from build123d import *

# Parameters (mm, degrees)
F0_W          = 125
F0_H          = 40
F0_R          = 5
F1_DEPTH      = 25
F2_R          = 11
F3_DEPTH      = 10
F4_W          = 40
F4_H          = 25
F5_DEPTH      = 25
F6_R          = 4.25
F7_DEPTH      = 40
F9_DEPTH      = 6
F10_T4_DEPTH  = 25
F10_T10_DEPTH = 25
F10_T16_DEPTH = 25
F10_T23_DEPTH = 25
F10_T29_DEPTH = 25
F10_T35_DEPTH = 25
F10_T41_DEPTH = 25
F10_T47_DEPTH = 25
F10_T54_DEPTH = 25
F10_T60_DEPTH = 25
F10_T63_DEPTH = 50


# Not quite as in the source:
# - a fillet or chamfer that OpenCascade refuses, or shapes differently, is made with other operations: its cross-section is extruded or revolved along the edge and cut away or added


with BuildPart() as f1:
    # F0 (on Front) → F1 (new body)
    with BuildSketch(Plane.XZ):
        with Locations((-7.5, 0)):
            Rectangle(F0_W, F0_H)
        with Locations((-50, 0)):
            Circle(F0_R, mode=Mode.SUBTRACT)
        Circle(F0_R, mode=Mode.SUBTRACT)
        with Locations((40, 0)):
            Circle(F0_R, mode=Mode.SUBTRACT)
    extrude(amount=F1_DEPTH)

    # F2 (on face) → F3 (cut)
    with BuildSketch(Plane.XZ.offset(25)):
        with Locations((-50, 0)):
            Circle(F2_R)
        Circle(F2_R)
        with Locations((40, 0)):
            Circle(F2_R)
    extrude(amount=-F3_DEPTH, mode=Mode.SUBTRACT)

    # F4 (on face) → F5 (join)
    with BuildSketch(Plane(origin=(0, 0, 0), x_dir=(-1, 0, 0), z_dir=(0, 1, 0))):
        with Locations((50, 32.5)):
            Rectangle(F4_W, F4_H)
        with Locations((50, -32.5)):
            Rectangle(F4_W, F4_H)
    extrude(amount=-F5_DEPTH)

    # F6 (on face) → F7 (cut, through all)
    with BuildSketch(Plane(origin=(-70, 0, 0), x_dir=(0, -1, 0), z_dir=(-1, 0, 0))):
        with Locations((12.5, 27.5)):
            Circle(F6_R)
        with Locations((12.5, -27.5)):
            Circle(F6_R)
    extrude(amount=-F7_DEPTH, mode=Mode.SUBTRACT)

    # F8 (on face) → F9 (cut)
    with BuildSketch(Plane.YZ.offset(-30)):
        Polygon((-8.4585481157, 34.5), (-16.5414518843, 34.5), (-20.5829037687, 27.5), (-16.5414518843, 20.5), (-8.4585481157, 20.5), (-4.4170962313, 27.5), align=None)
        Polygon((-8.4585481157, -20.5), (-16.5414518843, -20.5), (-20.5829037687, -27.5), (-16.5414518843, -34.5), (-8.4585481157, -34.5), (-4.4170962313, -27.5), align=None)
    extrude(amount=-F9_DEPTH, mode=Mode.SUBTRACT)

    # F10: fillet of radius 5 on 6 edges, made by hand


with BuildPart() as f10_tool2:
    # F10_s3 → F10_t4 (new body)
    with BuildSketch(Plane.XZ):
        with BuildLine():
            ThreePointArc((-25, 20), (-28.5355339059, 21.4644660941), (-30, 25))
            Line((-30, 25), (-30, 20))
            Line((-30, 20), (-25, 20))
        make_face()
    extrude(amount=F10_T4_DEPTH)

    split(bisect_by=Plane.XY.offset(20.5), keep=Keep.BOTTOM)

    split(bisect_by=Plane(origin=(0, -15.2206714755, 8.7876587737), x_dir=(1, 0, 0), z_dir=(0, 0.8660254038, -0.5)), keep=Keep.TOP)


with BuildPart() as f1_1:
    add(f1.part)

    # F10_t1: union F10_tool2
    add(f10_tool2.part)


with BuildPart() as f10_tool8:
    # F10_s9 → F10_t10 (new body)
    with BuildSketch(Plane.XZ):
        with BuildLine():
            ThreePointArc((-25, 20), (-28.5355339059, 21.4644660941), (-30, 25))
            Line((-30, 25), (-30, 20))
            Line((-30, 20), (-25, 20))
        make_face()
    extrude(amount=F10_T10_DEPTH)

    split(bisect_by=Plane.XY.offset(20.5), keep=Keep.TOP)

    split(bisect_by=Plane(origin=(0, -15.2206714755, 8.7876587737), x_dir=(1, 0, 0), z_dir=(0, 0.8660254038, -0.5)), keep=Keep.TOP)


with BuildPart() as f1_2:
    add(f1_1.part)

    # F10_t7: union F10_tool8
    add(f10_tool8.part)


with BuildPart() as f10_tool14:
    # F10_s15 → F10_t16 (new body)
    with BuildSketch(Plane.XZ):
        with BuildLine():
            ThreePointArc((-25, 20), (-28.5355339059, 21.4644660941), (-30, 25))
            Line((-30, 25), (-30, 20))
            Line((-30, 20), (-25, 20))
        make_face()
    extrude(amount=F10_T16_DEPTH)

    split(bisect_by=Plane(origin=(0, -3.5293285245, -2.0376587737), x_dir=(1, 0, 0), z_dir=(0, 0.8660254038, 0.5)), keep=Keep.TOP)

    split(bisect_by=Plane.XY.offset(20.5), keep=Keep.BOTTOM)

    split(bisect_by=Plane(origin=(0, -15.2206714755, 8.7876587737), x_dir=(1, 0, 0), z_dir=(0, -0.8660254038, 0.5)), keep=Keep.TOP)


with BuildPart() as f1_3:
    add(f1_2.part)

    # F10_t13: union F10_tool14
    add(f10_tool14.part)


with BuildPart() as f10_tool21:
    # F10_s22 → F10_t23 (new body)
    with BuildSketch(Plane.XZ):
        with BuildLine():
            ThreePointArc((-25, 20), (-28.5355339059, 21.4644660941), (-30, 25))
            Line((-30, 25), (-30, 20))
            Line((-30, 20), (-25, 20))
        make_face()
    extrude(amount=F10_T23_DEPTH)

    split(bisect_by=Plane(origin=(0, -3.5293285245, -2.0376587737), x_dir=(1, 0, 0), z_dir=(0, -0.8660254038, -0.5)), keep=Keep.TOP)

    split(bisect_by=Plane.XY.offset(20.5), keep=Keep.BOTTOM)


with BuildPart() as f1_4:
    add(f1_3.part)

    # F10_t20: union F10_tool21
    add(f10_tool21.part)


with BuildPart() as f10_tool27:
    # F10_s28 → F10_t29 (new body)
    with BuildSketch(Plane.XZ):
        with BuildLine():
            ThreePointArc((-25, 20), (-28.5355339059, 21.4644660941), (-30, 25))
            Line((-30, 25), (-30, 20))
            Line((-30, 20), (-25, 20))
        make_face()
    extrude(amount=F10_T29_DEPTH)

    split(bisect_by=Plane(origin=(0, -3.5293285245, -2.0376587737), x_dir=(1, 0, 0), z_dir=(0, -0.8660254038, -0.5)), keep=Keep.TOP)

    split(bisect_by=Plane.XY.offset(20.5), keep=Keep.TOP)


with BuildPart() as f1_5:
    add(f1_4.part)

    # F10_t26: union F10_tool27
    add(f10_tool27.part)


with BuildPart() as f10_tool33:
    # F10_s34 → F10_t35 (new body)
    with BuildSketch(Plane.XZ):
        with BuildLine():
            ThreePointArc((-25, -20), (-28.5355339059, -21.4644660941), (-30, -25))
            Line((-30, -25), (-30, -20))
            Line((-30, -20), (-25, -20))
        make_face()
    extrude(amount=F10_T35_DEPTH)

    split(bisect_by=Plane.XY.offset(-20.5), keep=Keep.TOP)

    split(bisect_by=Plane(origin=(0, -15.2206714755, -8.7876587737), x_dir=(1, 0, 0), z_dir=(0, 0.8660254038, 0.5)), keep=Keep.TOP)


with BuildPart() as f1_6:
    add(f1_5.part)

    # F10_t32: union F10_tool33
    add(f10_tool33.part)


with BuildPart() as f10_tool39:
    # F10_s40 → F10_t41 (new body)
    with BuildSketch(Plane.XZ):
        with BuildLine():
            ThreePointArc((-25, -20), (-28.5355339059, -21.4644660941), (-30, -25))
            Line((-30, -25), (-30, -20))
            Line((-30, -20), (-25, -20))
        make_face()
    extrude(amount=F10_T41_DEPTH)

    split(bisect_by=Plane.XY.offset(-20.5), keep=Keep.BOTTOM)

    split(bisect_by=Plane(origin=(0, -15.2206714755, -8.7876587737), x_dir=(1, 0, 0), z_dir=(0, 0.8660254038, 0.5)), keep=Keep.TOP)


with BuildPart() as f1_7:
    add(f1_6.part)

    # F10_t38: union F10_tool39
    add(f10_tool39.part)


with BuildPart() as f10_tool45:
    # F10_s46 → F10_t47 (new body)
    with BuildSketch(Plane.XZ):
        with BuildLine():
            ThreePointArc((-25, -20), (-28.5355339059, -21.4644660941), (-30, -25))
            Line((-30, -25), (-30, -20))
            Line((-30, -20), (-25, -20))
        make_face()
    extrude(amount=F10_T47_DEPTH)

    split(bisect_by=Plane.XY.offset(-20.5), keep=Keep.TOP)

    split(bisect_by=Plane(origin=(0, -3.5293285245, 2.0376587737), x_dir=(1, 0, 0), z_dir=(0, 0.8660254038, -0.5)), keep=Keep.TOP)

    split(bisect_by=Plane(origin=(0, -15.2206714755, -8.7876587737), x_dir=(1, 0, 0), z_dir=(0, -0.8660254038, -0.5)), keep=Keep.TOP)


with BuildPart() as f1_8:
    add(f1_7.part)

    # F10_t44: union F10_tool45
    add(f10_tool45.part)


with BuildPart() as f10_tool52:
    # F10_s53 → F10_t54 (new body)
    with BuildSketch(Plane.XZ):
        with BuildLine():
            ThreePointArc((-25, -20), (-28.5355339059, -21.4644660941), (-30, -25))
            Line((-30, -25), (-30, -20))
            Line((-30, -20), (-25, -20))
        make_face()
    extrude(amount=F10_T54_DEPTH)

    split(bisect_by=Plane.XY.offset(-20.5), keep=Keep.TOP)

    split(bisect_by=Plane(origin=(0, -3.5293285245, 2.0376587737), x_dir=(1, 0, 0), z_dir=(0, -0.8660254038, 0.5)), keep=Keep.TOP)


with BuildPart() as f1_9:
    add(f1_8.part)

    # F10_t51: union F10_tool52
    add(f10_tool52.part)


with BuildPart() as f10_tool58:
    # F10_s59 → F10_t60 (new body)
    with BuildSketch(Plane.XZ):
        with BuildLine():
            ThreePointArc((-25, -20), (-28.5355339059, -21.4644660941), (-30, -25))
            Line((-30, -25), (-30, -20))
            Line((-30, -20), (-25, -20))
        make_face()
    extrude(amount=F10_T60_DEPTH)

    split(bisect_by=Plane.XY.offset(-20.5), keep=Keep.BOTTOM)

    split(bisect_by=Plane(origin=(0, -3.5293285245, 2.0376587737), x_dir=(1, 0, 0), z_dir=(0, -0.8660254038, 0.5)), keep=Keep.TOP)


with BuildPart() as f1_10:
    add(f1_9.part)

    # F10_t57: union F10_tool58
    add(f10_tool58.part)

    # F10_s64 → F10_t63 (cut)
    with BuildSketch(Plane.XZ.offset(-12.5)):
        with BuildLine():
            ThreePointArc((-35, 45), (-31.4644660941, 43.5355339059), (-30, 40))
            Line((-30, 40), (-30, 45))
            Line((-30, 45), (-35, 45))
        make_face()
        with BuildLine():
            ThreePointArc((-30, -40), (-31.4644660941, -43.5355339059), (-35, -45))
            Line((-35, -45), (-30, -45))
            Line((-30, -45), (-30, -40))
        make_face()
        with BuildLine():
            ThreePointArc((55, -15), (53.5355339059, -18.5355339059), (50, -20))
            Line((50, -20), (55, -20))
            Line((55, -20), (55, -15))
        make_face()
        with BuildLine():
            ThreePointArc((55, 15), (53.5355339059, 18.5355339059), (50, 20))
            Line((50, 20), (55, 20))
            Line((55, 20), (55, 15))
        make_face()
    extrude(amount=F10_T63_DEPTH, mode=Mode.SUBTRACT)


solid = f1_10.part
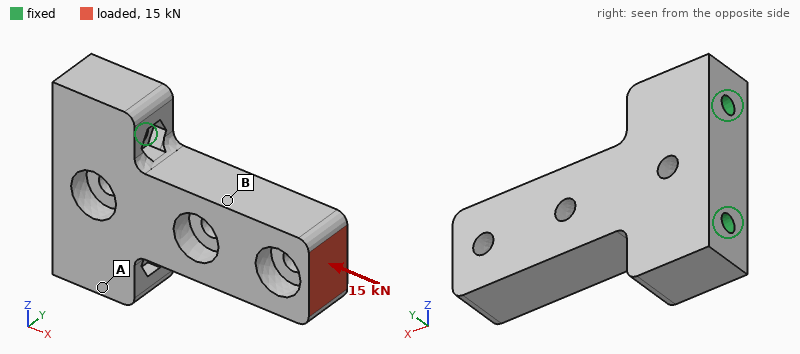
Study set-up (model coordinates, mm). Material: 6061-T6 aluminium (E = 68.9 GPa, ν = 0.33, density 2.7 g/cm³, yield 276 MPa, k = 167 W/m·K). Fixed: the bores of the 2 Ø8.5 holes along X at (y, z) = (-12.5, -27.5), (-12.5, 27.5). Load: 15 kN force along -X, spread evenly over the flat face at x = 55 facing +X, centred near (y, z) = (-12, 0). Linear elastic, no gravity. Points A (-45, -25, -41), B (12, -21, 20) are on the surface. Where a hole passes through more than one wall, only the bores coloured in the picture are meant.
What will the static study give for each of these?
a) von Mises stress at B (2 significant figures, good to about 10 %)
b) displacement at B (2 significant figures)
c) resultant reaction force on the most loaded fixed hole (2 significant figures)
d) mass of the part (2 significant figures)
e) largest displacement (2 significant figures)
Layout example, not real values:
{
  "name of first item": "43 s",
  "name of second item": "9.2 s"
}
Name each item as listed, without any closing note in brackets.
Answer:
{
  "von Mises stress at B": "29 MPa",
  "displacement at B": "22 µm",
  "resultant reaction force on the most loaded fixed hole": "8.0 kN",
  "mass of the part": "420 g",
  "largest displacement": "73 µm"
}
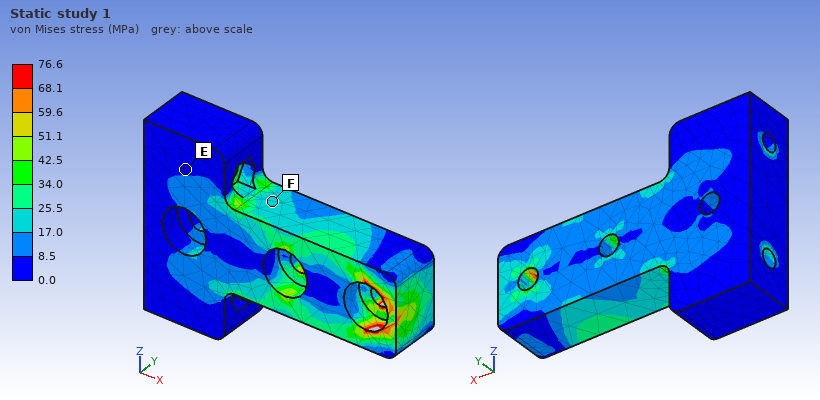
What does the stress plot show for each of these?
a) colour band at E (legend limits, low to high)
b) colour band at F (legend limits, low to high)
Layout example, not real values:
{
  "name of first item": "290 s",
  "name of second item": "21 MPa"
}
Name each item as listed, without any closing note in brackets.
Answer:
{
  "colour band at E": "0.0 to 8.5 MPa",
  "colour band at F": "17.0 to 25.5 MPa"
}
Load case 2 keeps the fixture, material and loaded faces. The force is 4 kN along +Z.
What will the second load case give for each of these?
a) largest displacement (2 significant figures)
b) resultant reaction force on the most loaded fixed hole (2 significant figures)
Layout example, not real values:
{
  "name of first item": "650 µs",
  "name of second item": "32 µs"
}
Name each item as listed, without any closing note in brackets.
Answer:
{
  "largest displacement": "0.17 mm",
  "resultant reaction force on the most loaded fixed hole": "8.3 kN"
}
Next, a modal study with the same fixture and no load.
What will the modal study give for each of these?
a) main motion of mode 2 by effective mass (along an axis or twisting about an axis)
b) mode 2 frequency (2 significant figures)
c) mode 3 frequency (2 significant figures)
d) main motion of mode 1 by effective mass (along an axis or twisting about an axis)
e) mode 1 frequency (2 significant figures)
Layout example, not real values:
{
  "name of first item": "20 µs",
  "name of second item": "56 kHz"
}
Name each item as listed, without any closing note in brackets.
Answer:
{
  "main motion of mode 2 by effective mass": "along Z",
  "mode 2 frequency": "3300 Hz",
  "mode 3 frequency": "6200 Hz",
  "main motion of mode 1 by effective mass": "along Y",
  "mode 1 frequency": "1800 Hz"
}
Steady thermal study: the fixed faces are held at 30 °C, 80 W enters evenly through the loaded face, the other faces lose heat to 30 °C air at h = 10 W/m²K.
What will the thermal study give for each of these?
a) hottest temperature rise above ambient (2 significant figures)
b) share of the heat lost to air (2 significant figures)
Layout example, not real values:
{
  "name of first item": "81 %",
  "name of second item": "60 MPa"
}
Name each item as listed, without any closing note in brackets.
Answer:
{
  "hottest temperature rise above ambient": "62 K",
  "share of the heat lost to air": "5.6 %"
}
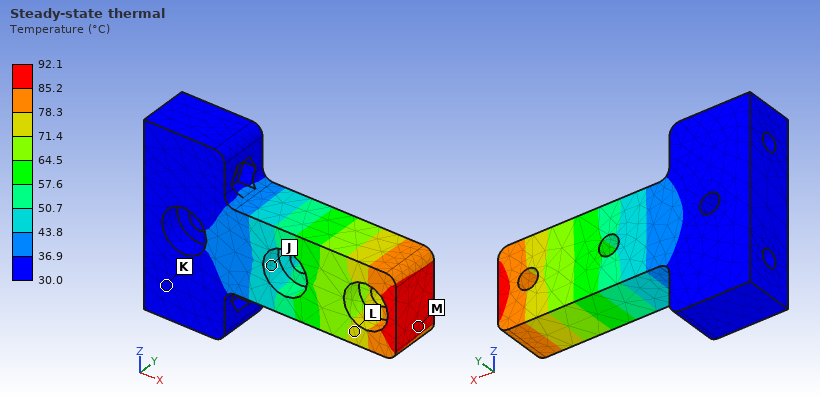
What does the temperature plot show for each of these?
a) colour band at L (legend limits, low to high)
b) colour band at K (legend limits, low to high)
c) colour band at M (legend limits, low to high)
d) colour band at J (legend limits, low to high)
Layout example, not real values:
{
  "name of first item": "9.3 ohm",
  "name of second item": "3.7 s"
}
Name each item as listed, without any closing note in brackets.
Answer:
{
  "colour band at L": "71.4 to 78.3 °C",
  "colour band at K": "30.0 to 36.9 °C",
  "colour band at M": "85.2 to 92.1 °C",
  "colour band at J": "43.8 to 50.7 °C"
}
